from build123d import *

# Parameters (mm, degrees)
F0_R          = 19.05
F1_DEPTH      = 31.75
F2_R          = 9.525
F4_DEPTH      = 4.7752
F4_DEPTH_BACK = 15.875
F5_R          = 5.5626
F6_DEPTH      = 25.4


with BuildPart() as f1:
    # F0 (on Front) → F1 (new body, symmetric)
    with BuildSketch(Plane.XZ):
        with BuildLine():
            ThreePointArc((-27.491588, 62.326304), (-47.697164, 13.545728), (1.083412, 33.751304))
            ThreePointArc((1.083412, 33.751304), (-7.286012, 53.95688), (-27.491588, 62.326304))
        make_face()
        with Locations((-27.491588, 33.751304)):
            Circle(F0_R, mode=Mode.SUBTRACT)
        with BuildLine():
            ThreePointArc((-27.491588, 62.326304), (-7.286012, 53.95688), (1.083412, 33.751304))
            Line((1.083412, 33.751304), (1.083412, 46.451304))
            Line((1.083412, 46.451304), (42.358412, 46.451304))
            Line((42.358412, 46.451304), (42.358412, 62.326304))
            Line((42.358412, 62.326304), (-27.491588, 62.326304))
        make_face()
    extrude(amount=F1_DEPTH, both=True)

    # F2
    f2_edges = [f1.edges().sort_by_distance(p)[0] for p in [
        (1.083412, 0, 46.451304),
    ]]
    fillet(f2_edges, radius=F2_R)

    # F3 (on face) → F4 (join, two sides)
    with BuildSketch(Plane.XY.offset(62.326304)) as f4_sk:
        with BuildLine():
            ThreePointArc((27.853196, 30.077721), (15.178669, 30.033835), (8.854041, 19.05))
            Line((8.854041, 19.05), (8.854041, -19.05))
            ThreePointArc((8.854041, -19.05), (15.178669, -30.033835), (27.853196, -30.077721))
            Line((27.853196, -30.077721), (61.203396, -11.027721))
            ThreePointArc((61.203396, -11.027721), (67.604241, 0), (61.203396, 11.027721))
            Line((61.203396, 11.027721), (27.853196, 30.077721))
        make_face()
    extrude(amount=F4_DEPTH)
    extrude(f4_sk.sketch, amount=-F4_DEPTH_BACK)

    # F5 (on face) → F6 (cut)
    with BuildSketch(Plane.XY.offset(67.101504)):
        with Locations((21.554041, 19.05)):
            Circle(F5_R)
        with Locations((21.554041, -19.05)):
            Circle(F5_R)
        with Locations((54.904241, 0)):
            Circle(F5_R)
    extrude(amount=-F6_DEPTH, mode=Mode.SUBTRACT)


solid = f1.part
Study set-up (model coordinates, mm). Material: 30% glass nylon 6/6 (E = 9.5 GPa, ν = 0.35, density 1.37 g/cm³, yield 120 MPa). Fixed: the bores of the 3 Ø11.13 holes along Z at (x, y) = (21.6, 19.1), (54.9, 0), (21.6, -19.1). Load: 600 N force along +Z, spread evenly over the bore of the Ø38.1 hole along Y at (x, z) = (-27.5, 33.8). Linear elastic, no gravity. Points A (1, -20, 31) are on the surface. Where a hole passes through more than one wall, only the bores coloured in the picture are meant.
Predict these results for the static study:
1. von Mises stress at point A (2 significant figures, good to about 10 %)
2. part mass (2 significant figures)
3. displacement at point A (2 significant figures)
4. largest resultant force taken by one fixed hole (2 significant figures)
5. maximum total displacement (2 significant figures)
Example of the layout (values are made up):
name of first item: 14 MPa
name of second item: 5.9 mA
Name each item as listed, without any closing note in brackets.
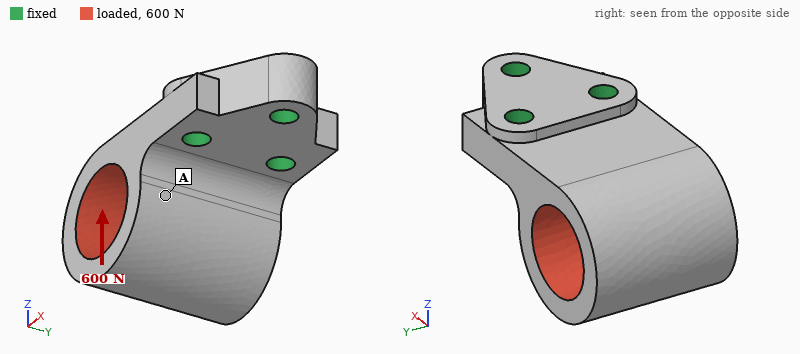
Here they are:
von Mises stress at point A: 1.7 MPa
part mass: 220 g
displacement at point A: 0.048 mm
largest resultant force taken by one fixed hole: 350 N
maximum total displacement: 0.17 mm
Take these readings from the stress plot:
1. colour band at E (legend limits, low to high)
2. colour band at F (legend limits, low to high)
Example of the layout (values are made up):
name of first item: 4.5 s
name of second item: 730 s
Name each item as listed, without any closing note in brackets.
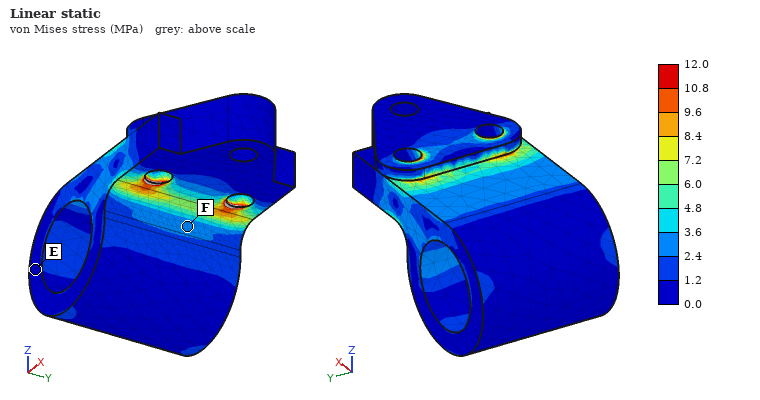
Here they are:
colour band at E: 0.0 to 1.2 MPa
colour band at F: 2.4 to 3.6 MPa
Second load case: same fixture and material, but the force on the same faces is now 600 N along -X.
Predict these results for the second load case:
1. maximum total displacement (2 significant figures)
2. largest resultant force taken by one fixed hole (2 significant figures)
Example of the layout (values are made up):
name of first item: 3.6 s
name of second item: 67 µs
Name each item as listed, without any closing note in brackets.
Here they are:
maximum total displacement: 0.11 mm
largest resultant force taken by one fixed hole: 290 N
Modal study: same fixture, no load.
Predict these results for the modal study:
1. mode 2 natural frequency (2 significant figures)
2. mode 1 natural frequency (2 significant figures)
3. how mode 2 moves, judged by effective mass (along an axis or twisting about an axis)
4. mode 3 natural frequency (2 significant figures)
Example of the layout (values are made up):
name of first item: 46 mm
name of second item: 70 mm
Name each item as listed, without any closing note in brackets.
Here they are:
mode 2 natural frequency: 2000 Hz
mode 1 natural frequency: 870 Hz
how mode 2 moves, judged by effective mass: along Y
mode 3 natural frequency: 3200 Hz
